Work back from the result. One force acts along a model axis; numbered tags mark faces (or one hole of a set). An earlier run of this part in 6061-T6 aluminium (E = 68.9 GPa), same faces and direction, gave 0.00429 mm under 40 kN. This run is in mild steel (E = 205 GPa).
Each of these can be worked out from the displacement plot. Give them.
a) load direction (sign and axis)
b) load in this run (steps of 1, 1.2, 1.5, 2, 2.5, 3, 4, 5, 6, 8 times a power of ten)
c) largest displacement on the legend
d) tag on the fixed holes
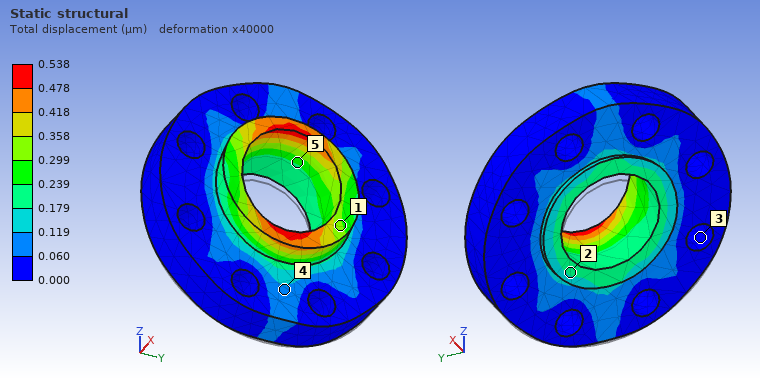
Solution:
+Z
15 kN
0.538 µm
3
